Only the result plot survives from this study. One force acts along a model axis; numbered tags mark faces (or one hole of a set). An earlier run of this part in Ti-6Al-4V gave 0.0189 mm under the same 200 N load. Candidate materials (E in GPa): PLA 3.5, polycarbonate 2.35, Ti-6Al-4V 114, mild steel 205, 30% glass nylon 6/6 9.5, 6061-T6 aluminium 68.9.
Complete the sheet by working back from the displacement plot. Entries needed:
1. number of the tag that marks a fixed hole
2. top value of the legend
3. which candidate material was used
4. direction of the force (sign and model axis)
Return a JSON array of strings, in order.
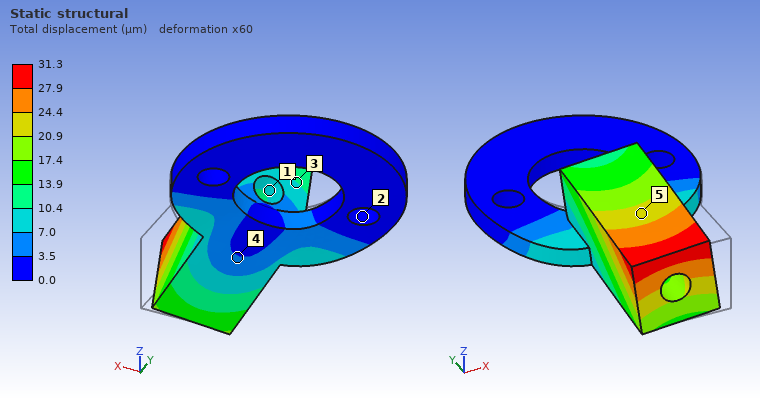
["2", "31.3 µm", "6061-T6 aluminium", "-X"]
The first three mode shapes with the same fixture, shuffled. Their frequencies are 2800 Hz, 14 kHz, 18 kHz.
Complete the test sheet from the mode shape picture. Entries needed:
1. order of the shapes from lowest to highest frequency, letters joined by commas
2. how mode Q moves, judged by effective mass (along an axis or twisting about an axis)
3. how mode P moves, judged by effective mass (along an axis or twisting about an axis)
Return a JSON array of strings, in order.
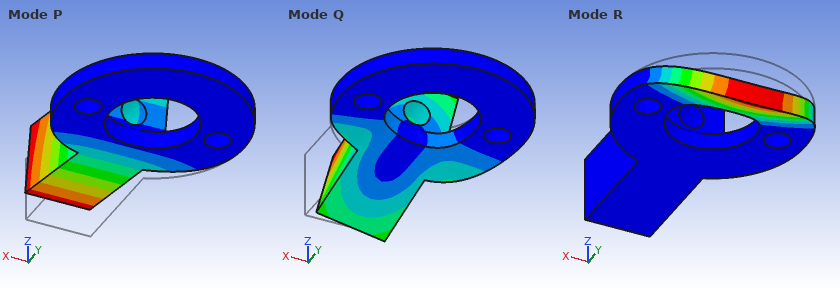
["P, Q, R", "along X", "along Z"]
